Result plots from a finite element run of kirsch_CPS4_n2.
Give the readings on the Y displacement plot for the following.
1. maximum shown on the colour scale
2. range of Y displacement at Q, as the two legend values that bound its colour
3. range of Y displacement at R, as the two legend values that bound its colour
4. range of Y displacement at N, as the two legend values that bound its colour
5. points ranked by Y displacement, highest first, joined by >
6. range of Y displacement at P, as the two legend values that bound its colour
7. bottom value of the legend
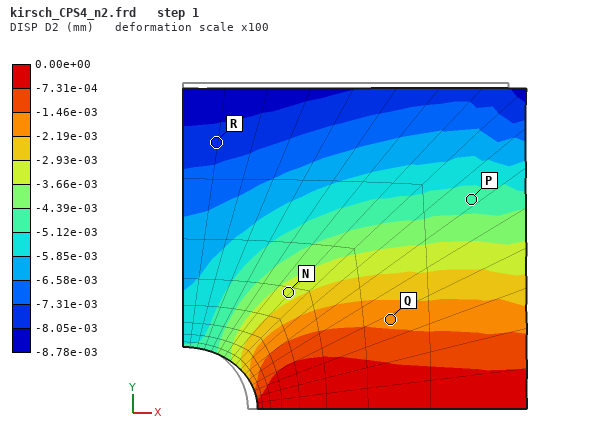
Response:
0.00e+00 mm
-2.19e-03 to -1.46e-03 mm
-8.05e-03 to -7.31e-03 mm
-3.66e-03 to -2.93e-03 mm
Q > N > P > R
-5.12e-03 to -4.39e-03 mm
-8.78e-03 mm
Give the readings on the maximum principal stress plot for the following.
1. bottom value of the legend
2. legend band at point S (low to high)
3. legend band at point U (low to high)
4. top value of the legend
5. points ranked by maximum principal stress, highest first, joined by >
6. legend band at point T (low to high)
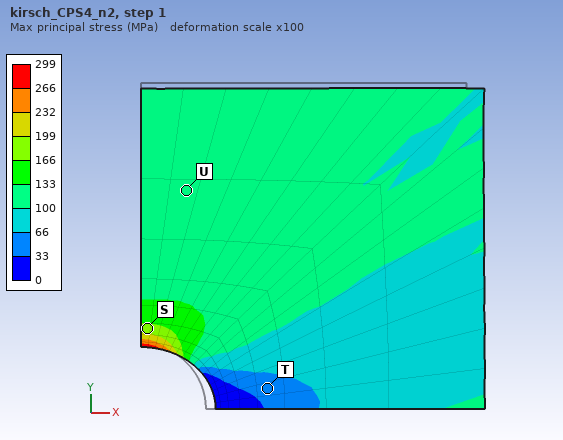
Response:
0 MPa
166 to 199 MPa
100 to 133 MPa
299 MPa
S > U > T
33 to 66 MPa
